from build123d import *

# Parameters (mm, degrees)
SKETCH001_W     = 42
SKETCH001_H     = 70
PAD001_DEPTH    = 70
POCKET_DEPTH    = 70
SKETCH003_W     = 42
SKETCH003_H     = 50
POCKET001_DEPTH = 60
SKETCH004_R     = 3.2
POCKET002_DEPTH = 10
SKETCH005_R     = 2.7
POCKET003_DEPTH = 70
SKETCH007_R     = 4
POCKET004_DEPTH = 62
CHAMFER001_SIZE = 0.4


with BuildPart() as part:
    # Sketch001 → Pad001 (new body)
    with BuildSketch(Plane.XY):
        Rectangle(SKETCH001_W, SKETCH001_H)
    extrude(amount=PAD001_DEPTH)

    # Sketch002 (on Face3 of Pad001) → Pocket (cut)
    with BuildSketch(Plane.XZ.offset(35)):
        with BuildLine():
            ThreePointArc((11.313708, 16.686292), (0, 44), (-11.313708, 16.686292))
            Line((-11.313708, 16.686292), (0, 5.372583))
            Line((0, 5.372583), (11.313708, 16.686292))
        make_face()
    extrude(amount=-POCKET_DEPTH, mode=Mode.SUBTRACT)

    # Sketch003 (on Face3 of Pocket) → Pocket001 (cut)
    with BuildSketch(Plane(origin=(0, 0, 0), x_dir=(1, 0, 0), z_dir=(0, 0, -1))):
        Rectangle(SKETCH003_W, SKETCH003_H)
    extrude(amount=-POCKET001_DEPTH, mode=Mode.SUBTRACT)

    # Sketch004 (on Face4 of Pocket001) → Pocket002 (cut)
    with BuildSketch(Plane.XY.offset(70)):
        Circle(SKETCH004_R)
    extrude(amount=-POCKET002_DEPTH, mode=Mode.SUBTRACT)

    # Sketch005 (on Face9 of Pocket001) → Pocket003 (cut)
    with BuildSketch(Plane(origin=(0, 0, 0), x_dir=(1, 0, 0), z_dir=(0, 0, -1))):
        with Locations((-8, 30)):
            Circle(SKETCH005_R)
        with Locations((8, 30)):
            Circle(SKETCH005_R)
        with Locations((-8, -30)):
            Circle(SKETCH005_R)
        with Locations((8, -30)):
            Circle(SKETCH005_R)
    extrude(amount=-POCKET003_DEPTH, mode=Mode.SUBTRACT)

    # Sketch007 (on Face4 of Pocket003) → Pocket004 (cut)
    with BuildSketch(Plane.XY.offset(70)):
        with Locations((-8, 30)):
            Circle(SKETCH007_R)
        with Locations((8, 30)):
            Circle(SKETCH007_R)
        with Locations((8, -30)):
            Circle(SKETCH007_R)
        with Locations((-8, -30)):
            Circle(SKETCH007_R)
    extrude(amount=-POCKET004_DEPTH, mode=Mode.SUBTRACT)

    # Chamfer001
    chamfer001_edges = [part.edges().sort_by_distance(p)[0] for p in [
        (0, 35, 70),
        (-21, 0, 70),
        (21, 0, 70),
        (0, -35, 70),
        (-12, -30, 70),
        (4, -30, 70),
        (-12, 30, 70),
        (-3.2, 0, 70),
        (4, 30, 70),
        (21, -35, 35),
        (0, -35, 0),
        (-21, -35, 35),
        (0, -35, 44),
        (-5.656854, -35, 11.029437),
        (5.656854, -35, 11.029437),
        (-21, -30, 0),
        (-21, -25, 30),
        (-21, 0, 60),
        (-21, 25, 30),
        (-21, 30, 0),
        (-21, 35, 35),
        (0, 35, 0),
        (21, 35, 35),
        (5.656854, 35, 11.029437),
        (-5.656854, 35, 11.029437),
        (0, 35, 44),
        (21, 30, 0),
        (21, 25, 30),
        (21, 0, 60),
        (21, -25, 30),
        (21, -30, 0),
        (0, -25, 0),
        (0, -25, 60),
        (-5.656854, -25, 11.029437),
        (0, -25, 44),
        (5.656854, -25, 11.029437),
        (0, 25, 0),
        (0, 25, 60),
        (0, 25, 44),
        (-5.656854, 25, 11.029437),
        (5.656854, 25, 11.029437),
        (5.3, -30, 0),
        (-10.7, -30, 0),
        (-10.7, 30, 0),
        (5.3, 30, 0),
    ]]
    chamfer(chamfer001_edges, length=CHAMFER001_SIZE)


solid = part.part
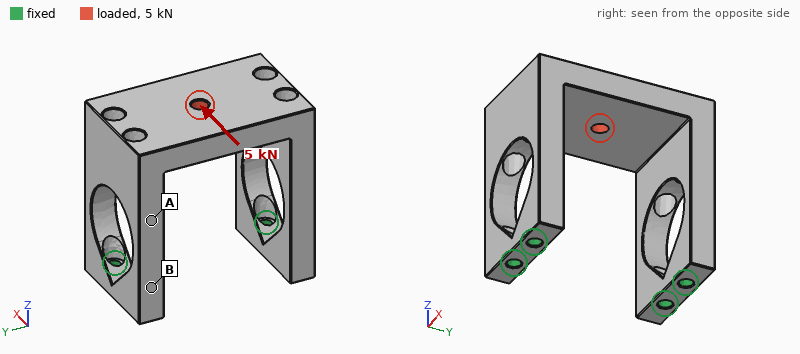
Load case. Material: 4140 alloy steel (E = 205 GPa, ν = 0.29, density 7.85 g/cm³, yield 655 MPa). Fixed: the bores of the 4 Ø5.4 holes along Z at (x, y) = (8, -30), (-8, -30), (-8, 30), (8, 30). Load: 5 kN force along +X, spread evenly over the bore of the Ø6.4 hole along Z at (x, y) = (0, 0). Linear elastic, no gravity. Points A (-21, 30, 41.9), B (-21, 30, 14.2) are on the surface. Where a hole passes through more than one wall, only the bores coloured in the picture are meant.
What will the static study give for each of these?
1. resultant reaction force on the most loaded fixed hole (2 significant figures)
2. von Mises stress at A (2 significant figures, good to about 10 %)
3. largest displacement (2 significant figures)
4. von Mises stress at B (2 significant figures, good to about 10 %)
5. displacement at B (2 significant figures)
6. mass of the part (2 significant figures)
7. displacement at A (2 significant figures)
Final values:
3.8 kN
55 MPa
0.17 mm
160 MPa
0.033 mm
430 g
0.12 mm
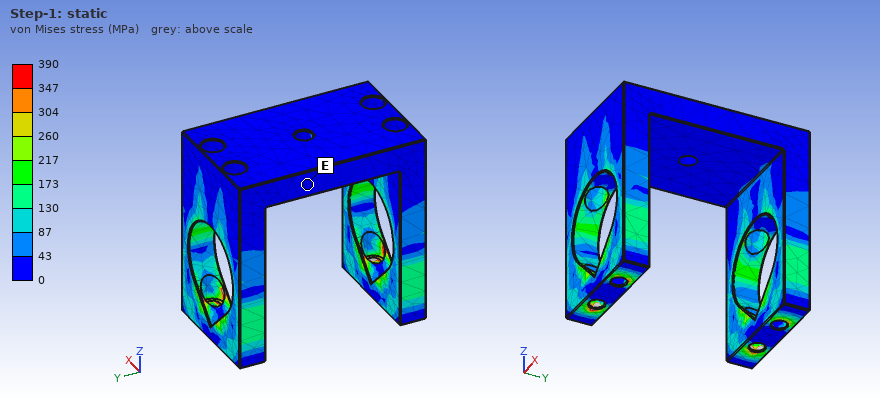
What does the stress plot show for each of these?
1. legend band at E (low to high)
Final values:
0 to 43 MPa
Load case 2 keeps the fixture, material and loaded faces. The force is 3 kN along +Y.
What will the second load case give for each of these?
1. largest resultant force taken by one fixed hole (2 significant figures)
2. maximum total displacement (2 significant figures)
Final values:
1.1 kN
0.12 mm
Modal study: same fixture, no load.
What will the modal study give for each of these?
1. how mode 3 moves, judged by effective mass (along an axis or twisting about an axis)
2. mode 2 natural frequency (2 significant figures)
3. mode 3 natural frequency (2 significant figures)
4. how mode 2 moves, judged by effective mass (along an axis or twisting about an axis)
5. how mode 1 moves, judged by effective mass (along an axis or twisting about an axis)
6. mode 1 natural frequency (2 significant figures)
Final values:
twisting about Z
1600 Hz
2400 Hz
along X
along Y
1500 Hz
